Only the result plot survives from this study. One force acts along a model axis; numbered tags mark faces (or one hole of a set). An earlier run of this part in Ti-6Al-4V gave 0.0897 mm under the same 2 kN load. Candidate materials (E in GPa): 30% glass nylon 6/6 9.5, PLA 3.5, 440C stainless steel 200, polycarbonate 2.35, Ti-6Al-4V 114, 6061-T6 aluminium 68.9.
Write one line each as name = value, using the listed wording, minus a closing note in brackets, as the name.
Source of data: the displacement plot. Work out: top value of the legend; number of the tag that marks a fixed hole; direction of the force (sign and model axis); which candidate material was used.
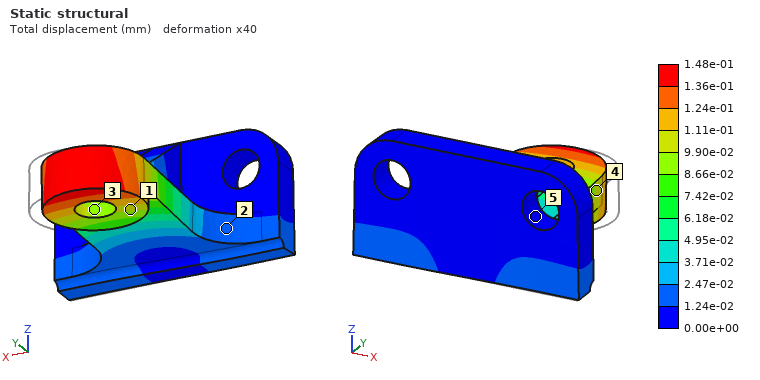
top value of the legend = 1.48e-01 mm
number of the tag that marks a fixed hole = 5
direction of the force = -X
which candidate material was used = 6061-T6 aluminium
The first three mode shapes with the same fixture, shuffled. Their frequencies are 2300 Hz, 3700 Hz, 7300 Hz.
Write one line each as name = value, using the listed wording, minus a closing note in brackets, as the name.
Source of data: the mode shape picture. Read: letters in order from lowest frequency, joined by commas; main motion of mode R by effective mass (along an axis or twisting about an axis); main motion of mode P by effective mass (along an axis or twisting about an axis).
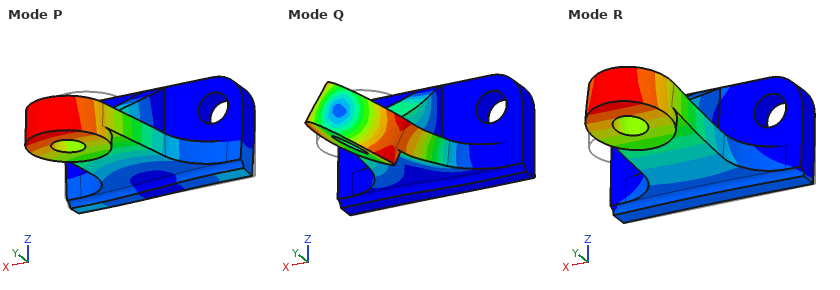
letters in order from lowest frequency, joined by commas = R, P, Q
main motion of mode R by effective mass = along Z
main motion of mode P by effective mass = along X
